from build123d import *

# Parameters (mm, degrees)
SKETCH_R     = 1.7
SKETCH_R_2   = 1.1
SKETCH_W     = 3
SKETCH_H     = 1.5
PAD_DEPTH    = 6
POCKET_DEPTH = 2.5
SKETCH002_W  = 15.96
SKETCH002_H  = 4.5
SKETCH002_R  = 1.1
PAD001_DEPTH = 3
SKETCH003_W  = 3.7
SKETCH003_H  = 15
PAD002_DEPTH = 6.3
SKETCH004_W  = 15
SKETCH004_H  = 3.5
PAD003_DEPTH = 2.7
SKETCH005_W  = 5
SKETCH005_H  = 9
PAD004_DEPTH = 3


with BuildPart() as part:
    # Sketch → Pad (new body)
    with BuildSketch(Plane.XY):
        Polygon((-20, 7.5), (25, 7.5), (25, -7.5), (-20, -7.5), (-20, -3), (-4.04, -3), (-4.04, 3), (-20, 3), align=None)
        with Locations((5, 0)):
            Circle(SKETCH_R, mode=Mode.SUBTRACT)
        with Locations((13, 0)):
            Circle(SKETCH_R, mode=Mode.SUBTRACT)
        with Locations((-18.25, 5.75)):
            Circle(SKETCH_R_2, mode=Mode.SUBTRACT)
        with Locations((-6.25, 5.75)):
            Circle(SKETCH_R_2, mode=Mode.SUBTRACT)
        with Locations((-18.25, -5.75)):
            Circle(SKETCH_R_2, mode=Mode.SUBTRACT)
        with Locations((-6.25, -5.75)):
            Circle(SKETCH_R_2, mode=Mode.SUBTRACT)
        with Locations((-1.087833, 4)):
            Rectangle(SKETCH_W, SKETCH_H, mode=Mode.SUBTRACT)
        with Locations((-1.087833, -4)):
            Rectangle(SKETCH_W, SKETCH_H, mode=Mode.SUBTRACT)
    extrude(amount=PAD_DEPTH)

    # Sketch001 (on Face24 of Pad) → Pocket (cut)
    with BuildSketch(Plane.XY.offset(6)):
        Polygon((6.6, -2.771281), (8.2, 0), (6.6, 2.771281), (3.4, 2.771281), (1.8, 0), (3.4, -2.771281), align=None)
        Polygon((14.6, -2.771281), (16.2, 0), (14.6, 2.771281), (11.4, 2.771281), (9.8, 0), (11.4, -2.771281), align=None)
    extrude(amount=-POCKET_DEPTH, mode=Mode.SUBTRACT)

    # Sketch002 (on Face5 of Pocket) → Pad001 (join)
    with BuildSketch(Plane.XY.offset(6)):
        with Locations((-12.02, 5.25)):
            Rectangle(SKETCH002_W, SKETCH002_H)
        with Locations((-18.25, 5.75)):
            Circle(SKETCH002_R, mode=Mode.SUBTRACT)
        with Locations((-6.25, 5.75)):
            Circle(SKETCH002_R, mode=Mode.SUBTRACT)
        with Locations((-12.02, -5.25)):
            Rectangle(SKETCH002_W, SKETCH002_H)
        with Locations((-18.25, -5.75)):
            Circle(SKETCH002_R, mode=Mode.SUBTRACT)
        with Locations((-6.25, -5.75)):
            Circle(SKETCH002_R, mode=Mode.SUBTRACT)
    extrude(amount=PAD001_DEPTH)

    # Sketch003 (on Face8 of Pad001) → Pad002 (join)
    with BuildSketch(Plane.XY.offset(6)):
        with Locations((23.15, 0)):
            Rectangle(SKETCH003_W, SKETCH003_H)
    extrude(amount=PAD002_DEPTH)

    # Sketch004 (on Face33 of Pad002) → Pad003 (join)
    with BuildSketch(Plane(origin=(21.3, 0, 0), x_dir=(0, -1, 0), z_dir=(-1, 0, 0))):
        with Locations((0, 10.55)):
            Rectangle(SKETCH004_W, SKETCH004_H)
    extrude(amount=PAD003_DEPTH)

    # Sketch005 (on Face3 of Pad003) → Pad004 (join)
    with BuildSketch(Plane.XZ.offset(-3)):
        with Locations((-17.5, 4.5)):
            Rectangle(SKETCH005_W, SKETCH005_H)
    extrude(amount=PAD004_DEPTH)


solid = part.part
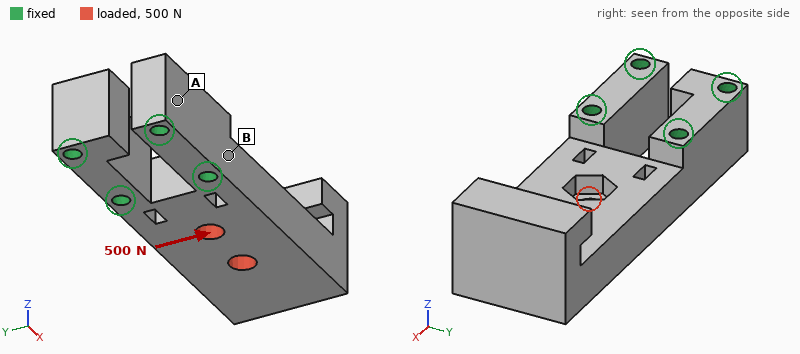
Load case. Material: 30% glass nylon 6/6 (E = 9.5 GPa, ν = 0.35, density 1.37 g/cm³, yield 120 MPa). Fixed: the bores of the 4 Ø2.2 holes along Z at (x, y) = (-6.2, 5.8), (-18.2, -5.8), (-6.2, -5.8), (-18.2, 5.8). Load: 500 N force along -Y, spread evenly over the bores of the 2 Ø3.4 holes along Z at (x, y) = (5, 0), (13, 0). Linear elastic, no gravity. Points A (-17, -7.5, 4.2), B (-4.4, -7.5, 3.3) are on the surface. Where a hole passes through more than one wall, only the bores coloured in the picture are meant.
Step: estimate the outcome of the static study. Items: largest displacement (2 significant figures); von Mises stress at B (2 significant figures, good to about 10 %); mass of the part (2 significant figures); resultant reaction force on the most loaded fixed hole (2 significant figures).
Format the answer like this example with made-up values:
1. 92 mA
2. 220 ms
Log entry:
1. 0.15 mm
2. 30 MPa
3. 5.7 g
4. 640 N
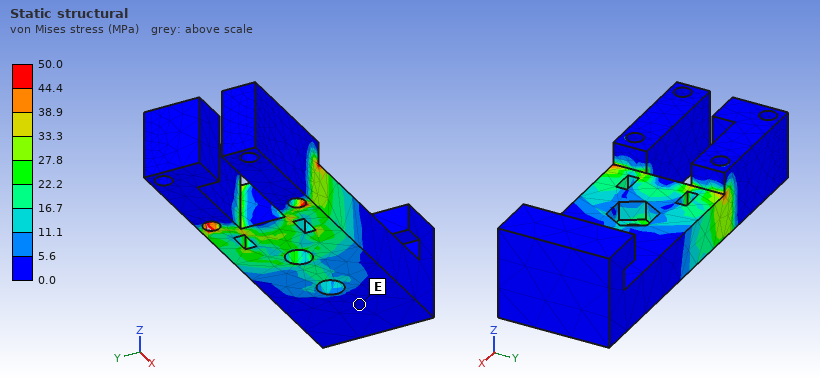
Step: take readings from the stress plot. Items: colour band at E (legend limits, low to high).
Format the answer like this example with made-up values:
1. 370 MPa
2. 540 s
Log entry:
1. 0.0 to 5.6 MPa
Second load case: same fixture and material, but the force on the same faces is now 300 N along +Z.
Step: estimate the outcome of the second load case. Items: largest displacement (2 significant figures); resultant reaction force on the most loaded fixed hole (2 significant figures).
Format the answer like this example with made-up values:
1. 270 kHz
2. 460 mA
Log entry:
1. 0.58 mm
2. 160 N
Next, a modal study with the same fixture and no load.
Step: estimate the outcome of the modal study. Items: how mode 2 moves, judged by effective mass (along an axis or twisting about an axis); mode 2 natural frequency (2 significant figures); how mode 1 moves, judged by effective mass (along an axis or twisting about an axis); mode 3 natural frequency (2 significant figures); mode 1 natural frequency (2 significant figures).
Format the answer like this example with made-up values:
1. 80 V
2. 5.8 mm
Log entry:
1. along Y
2. 3900 Hz
3. along Z
4. 6200 Hz
5. 1700 Hz
